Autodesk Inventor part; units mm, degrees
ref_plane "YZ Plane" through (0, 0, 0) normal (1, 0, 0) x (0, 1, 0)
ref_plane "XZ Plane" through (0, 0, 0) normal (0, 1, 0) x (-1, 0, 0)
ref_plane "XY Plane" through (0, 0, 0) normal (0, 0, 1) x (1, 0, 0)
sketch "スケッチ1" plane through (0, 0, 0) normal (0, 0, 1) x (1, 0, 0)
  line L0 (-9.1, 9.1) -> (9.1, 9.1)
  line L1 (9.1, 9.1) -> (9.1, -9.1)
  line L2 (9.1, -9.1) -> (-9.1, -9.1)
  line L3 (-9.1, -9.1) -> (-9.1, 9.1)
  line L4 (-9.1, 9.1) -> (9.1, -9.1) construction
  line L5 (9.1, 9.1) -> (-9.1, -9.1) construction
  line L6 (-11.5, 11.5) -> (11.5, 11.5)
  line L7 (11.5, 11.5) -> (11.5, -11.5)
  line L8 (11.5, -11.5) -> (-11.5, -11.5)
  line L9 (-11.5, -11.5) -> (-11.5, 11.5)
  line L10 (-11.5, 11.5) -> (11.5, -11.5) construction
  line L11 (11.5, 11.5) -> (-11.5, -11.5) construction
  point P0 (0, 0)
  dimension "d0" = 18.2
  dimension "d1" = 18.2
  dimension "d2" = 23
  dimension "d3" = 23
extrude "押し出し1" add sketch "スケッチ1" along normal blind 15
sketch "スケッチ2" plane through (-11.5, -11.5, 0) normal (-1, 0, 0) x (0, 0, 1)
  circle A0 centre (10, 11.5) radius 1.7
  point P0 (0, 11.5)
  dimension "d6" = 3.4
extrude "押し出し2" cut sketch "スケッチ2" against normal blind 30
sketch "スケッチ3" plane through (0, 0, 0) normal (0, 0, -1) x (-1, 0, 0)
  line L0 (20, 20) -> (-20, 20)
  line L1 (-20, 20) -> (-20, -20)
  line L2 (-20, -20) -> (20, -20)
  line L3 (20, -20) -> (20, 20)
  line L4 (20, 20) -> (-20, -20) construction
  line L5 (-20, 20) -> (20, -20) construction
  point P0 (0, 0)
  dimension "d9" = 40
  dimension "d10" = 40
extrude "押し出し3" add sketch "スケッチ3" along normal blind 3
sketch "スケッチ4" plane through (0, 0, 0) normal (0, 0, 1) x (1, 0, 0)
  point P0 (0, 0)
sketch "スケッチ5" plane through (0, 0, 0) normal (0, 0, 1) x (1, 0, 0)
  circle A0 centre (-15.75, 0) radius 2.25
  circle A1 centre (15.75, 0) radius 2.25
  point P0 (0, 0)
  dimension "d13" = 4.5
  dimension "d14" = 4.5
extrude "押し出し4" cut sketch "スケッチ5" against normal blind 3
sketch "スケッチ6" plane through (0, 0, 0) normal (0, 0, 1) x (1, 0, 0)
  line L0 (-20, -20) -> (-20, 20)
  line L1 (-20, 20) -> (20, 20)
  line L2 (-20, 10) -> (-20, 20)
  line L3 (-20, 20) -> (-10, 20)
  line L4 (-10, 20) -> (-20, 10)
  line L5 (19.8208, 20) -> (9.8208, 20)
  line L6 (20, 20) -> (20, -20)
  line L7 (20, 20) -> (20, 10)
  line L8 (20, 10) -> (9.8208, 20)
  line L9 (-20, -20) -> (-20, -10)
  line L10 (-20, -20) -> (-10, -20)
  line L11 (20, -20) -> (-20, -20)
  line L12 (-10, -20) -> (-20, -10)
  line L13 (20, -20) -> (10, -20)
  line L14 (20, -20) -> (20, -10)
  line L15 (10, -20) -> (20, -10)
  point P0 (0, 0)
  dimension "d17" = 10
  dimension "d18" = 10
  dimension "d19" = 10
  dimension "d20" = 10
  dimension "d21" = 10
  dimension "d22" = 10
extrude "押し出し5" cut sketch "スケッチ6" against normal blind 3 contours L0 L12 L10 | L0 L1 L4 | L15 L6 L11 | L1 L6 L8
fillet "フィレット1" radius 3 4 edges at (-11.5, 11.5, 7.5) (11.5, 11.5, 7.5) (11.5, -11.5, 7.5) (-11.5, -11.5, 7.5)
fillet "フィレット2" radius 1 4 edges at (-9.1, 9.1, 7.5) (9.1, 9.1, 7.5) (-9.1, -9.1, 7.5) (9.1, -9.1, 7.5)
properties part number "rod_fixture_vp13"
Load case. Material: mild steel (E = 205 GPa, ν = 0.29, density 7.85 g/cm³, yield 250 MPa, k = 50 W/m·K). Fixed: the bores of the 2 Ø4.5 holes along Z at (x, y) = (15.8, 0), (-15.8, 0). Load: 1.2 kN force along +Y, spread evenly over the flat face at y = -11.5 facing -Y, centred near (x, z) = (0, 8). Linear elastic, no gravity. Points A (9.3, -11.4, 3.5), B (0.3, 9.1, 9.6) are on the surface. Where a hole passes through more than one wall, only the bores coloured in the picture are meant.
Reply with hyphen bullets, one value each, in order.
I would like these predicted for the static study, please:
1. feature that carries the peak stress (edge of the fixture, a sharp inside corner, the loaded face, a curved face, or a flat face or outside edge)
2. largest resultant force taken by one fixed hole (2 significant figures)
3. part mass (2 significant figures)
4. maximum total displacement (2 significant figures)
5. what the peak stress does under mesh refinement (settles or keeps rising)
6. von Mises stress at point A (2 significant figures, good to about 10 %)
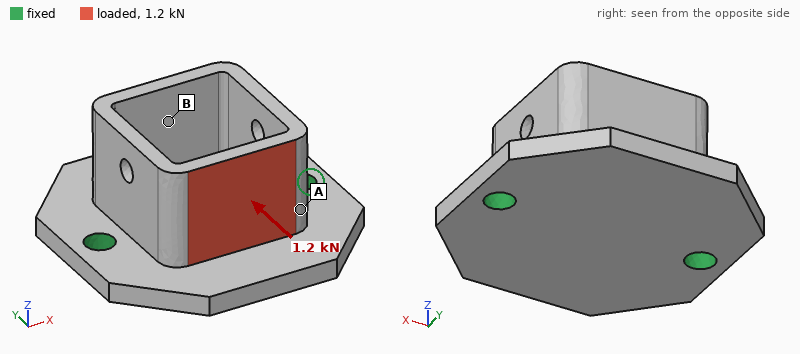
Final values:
- edge of the fixture
- 610 N
- 54 g
- 46 µm
- keeps rising
- 51 MPa
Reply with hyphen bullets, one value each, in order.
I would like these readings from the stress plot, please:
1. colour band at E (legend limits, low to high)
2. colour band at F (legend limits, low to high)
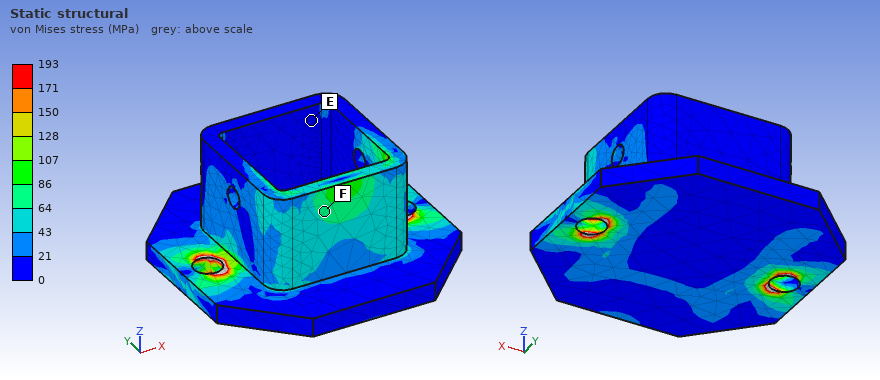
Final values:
- 0 to 21 MPa
- 64 to 86 MPa
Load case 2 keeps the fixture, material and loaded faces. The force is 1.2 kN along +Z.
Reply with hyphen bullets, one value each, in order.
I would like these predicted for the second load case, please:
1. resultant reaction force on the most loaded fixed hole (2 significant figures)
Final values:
- 620 N
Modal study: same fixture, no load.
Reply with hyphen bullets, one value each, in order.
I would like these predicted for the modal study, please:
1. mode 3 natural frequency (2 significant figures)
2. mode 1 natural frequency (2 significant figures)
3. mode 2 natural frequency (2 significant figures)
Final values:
- 13 kHz
- 5200 Hz
- 13 kHz
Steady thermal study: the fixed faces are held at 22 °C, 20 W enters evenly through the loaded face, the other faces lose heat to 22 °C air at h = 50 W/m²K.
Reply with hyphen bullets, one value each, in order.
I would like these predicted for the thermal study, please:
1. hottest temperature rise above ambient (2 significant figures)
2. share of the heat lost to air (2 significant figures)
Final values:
- 66 K
- 25 %
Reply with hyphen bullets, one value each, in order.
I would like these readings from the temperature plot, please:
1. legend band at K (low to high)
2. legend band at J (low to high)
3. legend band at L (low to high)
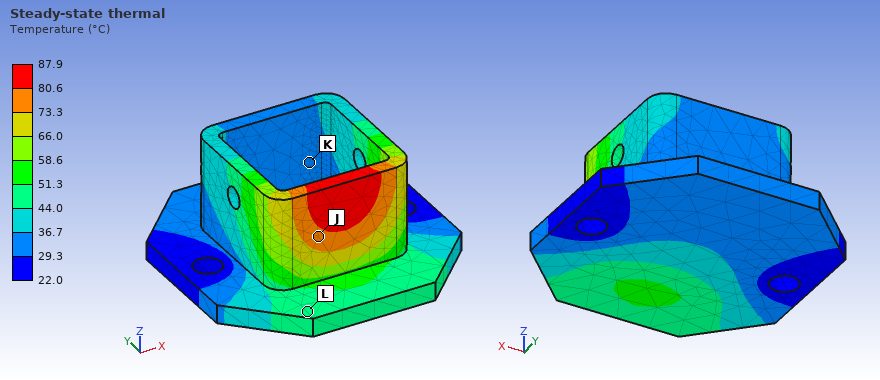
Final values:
- 29.3 to 36.7 °C
- 73.3 to 80.6 °C
- 44.0 to 51.3 °C
